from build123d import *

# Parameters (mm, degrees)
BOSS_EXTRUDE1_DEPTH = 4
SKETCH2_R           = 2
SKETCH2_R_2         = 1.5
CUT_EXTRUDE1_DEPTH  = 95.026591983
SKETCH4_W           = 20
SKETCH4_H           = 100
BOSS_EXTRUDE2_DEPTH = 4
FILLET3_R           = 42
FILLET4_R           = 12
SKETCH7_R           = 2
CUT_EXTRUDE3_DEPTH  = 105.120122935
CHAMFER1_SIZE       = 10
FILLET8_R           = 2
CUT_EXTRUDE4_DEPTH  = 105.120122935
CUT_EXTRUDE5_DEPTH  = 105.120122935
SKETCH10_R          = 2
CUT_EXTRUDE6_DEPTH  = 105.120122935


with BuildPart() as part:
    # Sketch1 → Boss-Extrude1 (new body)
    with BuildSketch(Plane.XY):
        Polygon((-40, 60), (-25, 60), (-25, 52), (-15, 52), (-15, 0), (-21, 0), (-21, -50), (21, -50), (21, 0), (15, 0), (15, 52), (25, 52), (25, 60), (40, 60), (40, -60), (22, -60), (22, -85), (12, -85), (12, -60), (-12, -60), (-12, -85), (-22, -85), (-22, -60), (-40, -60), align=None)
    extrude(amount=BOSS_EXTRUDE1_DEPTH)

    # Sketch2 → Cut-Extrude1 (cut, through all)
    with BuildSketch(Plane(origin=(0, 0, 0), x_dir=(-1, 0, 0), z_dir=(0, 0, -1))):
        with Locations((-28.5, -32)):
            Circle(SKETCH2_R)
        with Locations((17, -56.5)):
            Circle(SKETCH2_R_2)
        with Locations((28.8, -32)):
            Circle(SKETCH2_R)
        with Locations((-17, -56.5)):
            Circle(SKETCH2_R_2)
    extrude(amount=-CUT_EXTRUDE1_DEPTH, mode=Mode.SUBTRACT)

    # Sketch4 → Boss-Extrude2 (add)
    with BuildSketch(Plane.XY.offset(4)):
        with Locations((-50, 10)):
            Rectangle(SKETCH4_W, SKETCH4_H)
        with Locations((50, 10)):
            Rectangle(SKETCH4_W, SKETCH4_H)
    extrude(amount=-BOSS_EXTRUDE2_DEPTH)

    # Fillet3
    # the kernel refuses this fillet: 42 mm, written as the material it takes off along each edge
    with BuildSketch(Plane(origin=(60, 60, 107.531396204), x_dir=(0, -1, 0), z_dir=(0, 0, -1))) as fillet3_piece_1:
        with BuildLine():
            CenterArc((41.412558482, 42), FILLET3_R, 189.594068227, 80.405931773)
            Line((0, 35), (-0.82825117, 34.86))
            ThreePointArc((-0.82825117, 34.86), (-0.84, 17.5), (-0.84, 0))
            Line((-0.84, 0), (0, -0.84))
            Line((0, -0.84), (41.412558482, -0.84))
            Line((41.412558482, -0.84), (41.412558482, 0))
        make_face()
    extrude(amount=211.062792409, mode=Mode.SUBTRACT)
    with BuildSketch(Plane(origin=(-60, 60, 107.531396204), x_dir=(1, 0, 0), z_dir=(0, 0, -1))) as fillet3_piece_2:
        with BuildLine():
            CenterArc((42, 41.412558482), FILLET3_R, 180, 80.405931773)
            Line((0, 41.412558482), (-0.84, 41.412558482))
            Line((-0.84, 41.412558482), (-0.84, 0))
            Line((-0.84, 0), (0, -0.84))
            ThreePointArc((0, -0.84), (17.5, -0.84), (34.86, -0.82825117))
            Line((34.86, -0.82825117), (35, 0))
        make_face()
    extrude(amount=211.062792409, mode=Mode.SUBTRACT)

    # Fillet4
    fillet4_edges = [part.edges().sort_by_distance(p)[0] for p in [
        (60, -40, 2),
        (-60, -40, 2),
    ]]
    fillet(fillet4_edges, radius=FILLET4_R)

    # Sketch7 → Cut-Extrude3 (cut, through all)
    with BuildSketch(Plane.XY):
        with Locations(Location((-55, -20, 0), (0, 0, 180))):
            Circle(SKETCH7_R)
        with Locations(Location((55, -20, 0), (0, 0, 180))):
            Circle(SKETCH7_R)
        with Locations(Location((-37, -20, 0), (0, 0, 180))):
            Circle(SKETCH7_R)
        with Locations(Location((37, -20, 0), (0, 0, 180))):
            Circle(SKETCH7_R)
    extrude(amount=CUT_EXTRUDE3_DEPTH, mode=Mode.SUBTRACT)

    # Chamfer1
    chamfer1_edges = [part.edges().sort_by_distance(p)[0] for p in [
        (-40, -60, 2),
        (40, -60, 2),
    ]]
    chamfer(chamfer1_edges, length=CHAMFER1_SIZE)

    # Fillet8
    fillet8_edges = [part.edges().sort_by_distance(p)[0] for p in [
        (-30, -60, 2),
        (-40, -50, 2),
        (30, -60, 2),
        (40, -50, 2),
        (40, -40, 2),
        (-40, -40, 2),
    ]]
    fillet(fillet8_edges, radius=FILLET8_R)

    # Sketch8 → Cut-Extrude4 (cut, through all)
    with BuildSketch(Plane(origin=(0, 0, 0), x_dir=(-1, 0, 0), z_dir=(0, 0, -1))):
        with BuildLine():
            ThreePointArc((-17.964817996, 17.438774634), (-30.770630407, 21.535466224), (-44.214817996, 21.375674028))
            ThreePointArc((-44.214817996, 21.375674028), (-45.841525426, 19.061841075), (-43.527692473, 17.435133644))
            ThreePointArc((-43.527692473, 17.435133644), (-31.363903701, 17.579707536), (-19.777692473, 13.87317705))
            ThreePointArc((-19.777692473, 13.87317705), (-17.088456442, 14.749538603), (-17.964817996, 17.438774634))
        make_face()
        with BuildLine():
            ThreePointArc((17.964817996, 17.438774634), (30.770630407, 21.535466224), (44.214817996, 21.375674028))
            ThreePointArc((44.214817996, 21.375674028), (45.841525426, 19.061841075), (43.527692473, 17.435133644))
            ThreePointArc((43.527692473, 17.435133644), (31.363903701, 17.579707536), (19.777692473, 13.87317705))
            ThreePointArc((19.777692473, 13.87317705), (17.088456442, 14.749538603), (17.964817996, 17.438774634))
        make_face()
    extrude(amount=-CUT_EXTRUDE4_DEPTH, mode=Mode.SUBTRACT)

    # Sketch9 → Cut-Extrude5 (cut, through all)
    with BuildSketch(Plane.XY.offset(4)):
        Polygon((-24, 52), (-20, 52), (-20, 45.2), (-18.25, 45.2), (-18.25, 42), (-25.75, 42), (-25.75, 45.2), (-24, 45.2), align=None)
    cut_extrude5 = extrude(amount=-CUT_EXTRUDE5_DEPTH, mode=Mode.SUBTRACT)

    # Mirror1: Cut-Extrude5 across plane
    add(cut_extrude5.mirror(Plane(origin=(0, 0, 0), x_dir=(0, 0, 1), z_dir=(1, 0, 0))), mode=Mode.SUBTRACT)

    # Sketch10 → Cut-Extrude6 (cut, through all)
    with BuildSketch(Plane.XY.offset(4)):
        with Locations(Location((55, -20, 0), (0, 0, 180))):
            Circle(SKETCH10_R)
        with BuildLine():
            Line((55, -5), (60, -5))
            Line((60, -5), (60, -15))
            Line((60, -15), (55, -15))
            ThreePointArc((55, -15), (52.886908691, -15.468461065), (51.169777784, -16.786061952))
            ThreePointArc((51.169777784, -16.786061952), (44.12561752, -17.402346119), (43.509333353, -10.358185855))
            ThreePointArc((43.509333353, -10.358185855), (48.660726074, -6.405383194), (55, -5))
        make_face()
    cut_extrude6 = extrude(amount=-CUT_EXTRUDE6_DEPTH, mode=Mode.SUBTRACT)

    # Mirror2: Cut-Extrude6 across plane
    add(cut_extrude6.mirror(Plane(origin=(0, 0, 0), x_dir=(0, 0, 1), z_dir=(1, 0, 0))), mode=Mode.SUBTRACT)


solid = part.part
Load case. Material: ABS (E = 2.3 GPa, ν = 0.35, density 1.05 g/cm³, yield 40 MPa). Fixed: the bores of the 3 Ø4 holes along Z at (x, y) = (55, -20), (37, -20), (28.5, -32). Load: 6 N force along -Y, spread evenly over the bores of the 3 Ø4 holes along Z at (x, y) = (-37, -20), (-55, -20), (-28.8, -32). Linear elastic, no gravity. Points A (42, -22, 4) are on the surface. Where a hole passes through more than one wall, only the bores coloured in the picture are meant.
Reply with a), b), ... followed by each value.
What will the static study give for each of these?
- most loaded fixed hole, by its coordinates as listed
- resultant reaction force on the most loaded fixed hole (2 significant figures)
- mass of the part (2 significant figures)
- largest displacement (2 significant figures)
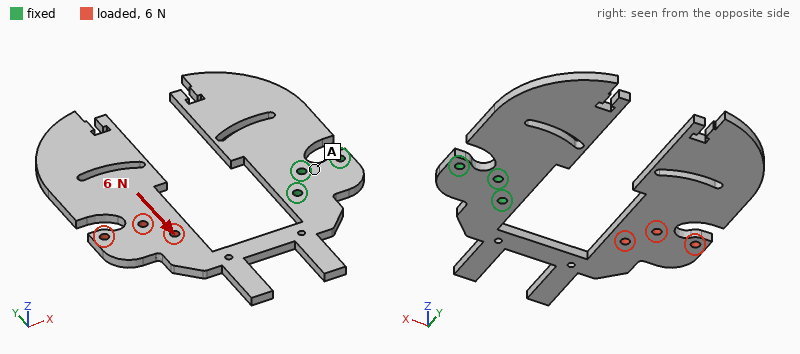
a) (28.5, -32)
b) 26 N
c) 35 g
d) 2.1 mm
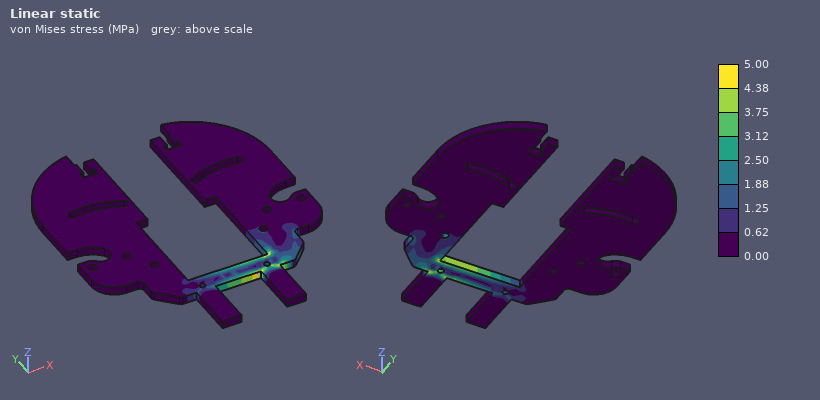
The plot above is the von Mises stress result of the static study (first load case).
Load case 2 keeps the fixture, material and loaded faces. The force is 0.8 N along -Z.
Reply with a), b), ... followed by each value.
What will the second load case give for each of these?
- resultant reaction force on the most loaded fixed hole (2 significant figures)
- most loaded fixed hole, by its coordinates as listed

a) 1.3 N
b) (28.5, -32)
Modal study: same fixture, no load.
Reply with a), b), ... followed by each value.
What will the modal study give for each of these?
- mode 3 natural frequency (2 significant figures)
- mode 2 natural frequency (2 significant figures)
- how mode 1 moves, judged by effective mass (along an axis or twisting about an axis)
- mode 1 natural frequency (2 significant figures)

a) 77 Hz
b) 63 Hz
c) along Z
d) 23 Hz
